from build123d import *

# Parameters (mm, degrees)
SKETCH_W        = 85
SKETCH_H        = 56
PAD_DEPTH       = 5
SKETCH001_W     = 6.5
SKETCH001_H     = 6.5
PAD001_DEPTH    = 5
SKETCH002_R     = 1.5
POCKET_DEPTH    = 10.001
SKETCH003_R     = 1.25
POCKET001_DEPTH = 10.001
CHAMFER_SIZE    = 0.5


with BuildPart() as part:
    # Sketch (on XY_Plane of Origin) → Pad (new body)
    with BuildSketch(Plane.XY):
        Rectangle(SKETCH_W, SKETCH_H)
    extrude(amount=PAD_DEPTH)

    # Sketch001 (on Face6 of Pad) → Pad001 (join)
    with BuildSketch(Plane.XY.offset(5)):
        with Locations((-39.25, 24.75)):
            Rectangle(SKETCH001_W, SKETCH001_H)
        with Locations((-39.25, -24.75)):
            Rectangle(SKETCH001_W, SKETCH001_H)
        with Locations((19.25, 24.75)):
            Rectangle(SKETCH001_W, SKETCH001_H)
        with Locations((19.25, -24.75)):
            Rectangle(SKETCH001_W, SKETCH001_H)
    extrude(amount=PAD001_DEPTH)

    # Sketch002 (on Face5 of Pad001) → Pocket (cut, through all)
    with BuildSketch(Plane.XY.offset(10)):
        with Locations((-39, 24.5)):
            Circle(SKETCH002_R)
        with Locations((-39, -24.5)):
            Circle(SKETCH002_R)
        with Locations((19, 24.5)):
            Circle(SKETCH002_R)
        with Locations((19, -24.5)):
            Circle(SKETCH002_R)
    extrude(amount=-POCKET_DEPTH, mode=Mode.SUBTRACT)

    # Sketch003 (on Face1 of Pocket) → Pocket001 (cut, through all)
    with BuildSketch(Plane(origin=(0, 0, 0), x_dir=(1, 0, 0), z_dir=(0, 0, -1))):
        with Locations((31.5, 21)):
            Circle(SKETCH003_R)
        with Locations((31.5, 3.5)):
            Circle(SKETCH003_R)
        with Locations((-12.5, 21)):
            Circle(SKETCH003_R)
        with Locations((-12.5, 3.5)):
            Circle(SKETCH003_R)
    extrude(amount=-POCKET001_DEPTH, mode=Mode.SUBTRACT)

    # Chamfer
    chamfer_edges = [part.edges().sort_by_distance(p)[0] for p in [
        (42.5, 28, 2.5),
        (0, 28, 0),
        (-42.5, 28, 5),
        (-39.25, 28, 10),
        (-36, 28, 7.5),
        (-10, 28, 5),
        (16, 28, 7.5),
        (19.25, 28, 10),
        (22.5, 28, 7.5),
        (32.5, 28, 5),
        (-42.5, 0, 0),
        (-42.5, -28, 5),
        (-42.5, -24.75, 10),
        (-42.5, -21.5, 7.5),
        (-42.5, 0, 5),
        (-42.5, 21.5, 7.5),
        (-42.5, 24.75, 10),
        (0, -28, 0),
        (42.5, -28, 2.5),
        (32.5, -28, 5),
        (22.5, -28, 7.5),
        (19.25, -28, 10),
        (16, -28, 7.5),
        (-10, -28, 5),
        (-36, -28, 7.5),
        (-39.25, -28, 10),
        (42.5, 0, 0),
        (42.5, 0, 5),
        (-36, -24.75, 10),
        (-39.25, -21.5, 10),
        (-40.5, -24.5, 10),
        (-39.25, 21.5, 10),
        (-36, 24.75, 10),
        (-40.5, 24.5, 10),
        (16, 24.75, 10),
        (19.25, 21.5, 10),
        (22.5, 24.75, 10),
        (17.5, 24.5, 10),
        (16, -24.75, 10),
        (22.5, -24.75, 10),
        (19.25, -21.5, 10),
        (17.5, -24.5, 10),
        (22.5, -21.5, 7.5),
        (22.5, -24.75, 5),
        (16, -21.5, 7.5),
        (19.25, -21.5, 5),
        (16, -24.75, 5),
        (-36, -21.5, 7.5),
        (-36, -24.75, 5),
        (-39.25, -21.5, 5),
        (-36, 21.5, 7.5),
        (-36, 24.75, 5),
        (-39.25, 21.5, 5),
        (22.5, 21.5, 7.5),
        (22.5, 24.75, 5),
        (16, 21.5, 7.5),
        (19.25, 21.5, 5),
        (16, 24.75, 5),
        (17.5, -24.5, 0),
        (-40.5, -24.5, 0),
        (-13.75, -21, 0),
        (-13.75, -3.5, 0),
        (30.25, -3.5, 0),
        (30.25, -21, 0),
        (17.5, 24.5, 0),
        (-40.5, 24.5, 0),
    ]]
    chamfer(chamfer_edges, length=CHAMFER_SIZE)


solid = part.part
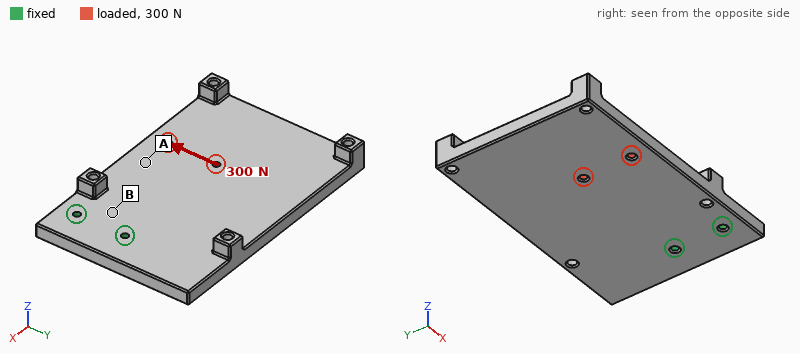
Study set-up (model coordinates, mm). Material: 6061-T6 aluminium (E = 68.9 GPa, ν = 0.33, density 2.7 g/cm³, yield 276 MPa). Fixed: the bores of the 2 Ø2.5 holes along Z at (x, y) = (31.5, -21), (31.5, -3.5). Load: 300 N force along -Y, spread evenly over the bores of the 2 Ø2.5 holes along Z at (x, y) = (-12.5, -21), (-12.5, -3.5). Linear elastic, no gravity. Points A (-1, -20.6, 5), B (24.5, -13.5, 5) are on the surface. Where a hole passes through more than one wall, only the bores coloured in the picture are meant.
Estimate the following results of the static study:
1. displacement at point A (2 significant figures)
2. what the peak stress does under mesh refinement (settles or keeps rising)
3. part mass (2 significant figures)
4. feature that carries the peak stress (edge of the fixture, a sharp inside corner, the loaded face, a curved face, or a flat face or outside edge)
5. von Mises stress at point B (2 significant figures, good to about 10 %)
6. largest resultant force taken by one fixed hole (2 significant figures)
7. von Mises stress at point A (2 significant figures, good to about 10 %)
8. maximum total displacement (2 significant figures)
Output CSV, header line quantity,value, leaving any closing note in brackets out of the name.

quantity,value
displacement at point A,10 µm
what the peak stress does under mesh refinement,keeps rising
part mass,65 g
feature that carries the peak stress,edge of the fixture
von Mises stress at point B,8.0 MPa
largest resultant force taken by one fixed hole,720 N
von Mises stress at point A,3.1 MPa
maximum total displacement,25 µm
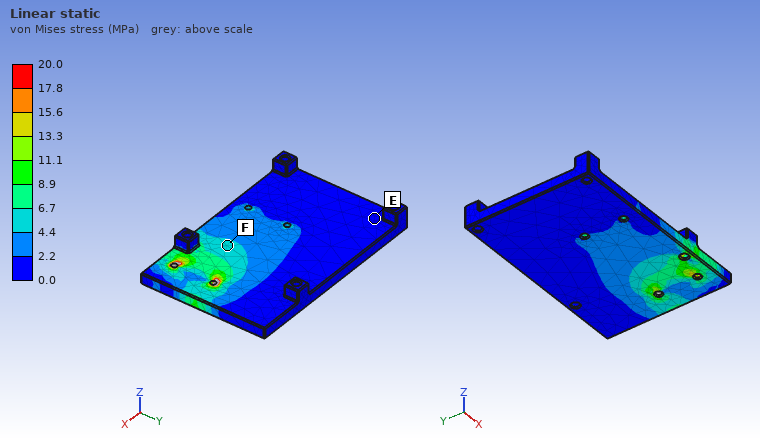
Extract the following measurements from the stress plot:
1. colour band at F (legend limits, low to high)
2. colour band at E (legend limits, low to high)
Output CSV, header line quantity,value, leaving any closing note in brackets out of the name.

quantity,value
colour band at F,4.4 to 6.7 MPa
colour band at E,0.0 to 2.2 MPa
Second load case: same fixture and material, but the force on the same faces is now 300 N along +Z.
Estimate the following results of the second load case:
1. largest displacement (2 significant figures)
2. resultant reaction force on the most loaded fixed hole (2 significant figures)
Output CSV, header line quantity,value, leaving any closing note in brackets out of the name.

quantity,value
largest displacement,0.61 mm
resultant reaction force on the most loaded fixed hole,150 N
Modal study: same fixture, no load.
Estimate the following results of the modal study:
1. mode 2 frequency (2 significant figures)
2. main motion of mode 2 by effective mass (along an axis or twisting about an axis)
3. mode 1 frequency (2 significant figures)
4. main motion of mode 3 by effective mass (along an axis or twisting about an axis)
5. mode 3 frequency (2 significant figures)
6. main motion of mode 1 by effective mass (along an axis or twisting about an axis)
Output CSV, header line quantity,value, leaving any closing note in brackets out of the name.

quantity,value
mode 2 frequency,1700 Hz
main motion of mode 2 by effective mass,twisting about X
mode 1 frequency,620 Hz
main motion of mode 3 by effective mass,along Y
mode 3 frequency,2900 Hz
main motion of mode 1 by effective mass,along Z
